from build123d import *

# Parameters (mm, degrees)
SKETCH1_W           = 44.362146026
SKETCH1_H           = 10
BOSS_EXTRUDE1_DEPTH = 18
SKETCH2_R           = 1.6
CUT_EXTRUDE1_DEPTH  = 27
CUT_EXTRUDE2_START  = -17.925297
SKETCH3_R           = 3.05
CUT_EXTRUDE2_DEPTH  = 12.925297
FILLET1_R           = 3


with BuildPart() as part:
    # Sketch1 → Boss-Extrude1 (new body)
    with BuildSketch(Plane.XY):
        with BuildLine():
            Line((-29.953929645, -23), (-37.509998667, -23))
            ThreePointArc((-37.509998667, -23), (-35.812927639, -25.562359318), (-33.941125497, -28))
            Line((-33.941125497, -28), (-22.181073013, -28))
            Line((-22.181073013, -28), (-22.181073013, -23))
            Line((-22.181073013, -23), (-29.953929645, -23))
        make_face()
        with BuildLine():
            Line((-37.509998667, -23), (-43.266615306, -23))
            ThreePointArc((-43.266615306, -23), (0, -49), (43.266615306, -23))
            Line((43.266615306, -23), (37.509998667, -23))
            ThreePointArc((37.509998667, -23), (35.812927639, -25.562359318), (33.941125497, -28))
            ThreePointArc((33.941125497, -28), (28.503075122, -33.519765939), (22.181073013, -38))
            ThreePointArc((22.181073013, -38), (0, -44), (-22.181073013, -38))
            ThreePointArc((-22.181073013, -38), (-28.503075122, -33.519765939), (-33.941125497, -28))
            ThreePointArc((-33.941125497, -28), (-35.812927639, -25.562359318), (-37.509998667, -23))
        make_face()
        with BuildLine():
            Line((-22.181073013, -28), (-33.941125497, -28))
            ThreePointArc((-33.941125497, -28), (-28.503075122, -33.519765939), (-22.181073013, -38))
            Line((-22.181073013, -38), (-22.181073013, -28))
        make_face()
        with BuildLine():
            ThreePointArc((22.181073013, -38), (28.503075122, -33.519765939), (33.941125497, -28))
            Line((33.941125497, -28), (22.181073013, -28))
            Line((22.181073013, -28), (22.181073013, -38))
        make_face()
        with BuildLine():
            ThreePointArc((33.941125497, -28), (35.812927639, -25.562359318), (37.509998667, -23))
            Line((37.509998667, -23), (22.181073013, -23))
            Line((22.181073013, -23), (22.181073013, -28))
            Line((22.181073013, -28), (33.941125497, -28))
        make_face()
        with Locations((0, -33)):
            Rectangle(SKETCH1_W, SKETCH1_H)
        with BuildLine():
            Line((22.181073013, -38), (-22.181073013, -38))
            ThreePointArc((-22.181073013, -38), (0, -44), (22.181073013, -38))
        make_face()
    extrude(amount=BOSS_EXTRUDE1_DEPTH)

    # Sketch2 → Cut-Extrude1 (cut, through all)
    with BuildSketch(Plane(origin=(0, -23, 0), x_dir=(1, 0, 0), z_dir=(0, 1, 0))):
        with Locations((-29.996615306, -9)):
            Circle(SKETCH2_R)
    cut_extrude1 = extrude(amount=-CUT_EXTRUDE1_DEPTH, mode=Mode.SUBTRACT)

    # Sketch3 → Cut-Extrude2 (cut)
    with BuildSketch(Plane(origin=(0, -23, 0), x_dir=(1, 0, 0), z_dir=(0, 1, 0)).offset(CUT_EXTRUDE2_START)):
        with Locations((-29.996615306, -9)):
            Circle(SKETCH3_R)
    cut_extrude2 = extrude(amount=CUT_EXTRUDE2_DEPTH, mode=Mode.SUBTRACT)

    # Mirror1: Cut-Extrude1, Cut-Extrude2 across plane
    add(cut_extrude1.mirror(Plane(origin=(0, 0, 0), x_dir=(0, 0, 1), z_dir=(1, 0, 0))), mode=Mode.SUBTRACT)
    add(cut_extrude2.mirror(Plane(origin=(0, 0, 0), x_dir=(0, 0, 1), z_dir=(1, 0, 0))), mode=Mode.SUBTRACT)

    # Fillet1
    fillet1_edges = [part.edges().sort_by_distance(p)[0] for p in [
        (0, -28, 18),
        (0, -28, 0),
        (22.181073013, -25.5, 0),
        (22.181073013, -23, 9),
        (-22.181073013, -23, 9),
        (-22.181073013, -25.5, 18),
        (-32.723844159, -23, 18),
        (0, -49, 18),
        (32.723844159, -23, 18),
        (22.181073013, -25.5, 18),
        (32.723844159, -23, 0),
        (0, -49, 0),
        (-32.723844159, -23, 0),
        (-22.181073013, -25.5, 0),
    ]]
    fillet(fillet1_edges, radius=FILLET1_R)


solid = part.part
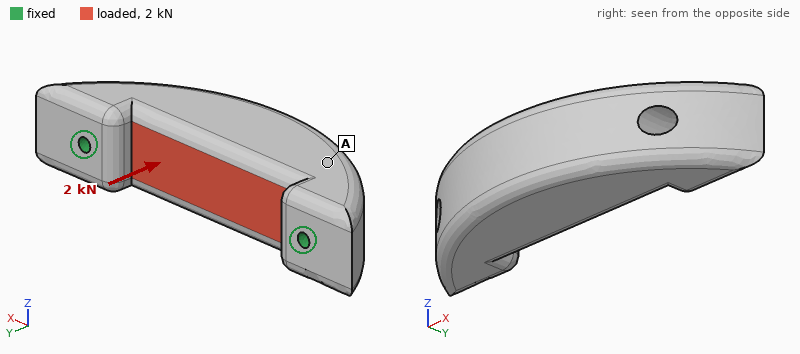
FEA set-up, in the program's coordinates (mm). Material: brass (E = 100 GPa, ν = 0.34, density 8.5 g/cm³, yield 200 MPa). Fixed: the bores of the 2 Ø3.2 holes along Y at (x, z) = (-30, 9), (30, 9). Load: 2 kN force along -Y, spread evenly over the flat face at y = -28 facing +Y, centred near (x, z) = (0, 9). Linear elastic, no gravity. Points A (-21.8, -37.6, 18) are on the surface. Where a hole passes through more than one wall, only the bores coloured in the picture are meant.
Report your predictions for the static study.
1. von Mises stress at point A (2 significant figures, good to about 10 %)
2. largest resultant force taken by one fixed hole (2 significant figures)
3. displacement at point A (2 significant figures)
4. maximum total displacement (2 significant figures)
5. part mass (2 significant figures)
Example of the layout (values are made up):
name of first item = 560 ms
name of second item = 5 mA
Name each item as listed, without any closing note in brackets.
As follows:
von Mises stress at point A = 6.3 MPa
largest resultant force taken by one fixed hole = 1.2 kN
displacement at point A = 2.9 µm
maximum total displacement = 5.3 µm
part mass = 200 g
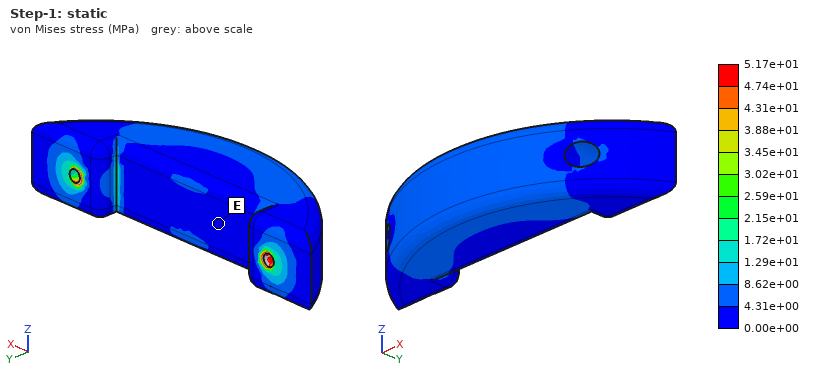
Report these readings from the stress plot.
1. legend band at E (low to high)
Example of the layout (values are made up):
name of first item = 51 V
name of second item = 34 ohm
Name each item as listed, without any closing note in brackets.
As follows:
legend band at E = 0.00e+00 to 4.31e+00 MPa
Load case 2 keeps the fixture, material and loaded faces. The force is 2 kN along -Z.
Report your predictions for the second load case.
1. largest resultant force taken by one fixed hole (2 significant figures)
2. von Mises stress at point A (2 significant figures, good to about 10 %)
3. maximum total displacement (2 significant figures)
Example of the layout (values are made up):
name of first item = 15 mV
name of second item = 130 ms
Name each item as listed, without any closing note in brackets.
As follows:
largest resultant force taken by one fixed hole = 1.0 kN
von Mises stress at point A = 12 MPa
maximum total displacement = 16 µm
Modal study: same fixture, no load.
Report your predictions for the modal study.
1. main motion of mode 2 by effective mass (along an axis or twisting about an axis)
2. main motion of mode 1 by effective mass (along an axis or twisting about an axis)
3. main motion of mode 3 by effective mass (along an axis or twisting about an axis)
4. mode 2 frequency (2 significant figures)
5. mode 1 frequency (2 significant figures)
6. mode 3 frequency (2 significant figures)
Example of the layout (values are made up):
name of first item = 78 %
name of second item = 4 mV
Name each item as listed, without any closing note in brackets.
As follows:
main motion of mode 2 by effective mass = along Y
main motion of mode 1 by effective mass = along Z
main motion of mode 3 by effective mass = along X
mode 2 frequency = 9000 Hz
mode 1 frequency = 3000 Hz
mode 3 frequency = 10 kHz
